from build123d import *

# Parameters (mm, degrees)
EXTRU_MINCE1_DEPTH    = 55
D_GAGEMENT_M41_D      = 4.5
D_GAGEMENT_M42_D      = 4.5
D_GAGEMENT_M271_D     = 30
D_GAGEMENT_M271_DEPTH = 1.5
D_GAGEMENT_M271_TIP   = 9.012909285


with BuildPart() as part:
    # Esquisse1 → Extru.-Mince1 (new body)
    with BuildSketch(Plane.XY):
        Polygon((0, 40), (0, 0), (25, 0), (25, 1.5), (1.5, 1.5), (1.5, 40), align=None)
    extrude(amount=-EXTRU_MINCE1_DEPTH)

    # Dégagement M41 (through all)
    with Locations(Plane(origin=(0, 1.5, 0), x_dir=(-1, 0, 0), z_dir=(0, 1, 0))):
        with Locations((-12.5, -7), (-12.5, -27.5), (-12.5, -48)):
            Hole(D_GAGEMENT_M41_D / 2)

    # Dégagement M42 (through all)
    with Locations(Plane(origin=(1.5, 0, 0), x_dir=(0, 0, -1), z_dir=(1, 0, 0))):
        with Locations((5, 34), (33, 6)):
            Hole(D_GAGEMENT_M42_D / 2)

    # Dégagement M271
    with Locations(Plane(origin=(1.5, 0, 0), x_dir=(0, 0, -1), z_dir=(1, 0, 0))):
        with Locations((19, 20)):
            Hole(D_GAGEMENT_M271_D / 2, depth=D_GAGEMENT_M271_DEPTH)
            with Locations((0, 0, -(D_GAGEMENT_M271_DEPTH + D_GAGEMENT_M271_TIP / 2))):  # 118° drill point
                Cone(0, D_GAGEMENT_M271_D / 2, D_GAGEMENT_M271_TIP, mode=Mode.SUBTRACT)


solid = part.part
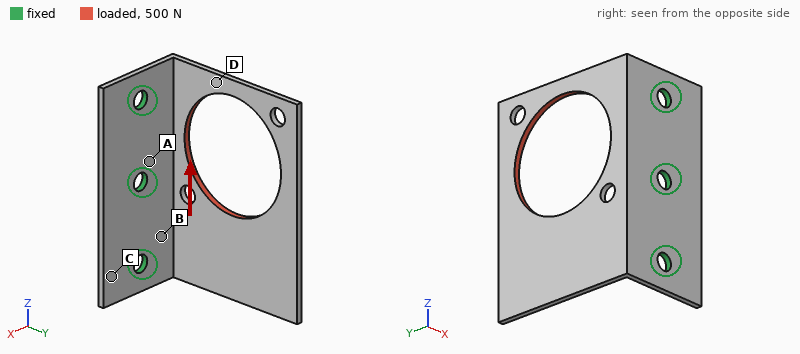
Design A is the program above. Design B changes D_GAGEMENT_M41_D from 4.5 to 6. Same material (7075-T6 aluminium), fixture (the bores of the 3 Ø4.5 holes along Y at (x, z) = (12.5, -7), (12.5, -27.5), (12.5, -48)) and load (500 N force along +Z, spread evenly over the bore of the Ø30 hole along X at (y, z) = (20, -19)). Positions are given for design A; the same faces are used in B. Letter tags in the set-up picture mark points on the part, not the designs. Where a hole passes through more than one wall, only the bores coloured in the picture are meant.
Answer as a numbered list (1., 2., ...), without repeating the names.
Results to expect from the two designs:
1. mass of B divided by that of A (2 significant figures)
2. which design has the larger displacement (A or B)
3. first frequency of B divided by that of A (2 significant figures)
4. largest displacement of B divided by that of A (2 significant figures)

1. 0.99
2. A
3. 1.0
4. 0.87
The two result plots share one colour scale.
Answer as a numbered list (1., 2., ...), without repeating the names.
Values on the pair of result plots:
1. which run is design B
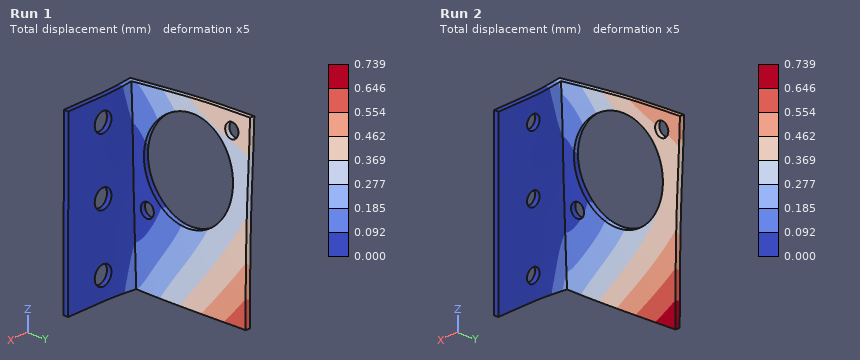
1. Run 1
